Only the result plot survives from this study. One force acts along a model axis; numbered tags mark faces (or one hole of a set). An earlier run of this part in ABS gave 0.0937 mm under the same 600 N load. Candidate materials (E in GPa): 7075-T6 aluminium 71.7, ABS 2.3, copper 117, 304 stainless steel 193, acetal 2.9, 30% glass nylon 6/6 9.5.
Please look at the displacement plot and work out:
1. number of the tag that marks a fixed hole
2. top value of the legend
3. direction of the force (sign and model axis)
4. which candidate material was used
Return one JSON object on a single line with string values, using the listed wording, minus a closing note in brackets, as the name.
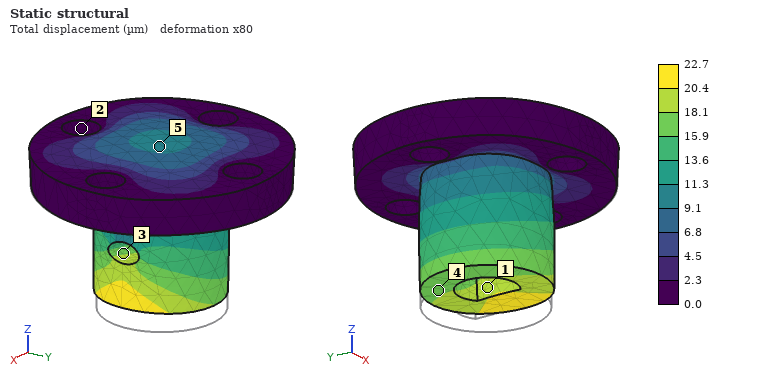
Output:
{"number of the tag that marks a fixed hole": "2", "top value of the legend": "22.7 µm", "direction of the force": "+Z", "which candidate material was used": "30% glass nylon 6/6"}
